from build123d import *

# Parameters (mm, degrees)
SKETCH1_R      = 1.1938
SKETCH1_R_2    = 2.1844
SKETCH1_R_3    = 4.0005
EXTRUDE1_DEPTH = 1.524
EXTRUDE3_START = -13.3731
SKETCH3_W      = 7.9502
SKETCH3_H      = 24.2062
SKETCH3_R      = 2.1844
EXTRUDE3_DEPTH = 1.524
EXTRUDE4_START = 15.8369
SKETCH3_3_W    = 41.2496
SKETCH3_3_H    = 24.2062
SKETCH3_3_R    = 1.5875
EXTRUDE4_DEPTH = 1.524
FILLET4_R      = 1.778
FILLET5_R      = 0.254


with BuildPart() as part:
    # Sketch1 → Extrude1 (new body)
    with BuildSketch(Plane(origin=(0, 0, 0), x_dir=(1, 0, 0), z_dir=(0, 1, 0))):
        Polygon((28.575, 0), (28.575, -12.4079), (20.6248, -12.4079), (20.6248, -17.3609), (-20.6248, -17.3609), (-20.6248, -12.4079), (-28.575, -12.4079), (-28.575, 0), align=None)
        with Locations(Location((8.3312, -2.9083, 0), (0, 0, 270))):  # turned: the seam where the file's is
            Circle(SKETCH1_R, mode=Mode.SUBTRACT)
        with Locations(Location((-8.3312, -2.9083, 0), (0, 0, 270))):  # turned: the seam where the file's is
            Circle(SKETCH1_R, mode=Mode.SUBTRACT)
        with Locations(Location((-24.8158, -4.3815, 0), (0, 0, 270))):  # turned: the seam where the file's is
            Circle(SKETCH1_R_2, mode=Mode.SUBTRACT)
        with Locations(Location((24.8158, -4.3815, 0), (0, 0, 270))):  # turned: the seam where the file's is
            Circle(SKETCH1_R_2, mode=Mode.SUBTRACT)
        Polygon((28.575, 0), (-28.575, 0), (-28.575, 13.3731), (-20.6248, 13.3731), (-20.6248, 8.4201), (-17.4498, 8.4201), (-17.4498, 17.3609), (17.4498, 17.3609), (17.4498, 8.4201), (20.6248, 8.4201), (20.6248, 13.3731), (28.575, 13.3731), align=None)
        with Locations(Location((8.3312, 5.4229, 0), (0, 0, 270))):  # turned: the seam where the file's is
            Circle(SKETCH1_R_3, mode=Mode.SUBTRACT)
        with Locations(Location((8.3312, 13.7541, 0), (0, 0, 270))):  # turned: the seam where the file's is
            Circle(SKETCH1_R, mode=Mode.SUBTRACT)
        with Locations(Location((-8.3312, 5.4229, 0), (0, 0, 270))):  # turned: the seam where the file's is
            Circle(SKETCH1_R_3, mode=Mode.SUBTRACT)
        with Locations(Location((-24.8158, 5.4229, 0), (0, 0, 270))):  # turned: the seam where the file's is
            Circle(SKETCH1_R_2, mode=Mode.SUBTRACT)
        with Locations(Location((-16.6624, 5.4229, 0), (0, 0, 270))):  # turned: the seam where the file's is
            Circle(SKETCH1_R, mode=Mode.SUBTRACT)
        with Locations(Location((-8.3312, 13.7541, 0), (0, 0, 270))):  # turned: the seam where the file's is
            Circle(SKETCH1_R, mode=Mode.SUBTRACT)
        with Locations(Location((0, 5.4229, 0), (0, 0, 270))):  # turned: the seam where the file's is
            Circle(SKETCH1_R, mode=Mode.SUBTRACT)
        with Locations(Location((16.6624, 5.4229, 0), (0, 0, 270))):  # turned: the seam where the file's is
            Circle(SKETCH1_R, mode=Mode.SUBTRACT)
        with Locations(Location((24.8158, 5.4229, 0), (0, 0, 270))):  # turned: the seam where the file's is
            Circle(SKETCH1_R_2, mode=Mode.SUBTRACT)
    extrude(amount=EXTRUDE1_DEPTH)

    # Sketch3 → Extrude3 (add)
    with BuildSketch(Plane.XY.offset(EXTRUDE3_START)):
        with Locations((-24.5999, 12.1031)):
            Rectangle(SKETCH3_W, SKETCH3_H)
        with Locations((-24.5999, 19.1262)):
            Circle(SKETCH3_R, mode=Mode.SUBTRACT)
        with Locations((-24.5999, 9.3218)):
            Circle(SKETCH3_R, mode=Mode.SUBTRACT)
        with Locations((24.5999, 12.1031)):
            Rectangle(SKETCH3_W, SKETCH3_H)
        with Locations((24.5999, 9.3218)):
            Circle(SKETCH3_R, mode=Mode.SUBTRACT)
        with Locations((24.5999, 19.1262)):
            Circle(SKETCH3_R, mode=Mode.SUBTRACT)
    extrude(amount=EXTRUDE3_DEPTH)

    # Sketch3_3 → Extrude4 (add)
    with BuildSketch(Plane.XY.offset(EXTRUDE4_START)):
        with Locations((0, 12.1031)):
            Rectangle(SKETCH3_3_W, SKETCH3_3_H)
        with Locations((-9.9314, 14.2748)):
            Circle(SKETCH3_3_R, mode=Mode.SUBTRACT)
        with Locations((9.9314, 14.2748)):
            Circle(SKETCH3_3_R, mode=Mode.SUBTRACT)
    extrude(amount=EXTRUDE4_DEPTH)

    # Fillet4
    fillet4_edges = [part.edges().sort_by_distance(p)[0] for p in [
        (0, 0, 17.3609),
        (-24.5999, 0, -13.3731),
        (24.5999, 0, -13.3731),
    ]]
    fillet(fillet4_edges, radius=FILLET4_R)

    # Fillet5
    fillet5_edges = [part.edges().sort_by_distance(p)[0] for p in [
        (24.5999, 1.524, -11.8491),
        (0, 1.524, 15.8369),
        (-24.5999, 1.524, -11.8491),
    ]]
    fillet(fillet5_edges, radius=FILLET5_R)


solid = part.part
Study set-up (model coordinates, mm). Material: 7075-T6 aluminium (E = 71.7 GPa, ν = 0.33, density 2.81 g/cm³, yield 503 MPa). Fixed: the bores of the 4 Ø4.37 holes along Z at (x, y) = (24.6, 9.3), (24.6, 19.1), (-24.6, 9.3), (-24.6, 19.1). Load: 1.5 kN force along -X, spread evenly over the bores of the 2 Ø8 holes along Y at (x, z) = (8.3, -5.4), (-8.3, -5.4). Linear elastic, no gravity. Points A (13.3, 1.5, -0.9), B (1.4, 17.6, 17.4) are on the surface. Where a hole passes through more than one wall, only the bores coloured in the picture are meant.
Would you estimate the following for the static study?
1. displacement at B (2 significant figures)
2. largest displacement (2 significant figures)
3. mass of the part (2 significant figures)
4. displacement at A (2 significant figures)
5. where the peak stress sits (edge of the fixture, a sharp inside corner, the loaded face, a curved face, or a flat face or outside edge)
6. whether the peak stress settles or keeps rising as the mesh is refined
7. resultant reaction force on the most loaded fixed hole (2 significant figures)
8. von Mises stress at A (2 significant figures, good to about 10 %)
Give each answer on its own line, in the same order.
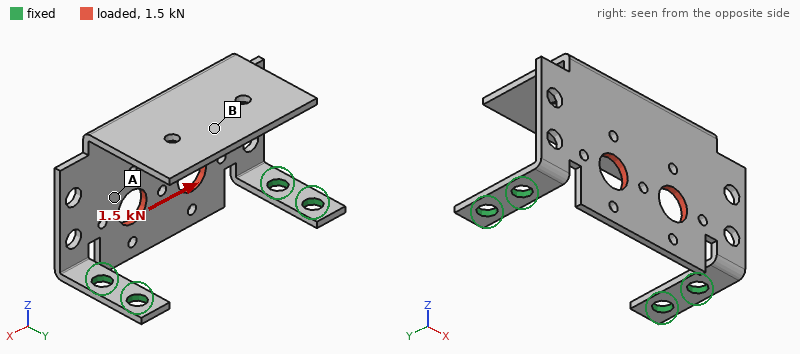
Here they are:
0.36 mm
0.45 mm
12 g
0.18 mm
a sharp inside corner
keeps rising
850 N
68 MPa
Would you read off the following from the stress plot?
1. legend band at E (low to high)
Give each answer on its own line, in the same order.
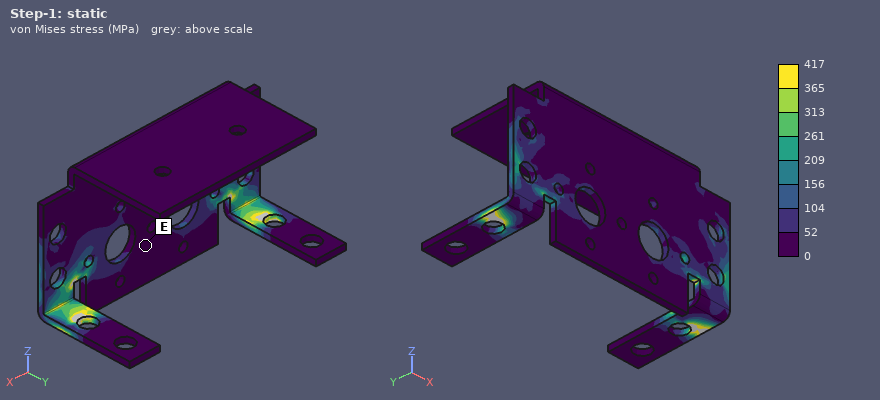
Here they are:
0 to 52 MPa
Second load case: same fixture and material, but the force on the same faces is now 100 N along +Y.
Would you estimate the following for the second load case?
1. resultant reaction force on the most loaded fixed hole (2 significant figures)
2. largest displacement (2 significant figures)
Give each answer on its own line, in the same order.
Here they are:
50 N
0.80 mm
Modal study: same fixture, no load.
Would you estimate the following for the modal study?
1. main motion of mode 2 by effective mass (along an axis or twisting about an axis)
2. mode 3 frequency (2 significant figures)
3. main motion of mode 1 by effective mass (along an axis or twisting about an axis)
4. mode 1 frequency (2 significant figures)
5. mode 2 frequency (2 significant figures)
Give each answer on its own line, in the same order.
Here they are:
along X
1300 Hz
along Y
310 Hz
990 Hz
